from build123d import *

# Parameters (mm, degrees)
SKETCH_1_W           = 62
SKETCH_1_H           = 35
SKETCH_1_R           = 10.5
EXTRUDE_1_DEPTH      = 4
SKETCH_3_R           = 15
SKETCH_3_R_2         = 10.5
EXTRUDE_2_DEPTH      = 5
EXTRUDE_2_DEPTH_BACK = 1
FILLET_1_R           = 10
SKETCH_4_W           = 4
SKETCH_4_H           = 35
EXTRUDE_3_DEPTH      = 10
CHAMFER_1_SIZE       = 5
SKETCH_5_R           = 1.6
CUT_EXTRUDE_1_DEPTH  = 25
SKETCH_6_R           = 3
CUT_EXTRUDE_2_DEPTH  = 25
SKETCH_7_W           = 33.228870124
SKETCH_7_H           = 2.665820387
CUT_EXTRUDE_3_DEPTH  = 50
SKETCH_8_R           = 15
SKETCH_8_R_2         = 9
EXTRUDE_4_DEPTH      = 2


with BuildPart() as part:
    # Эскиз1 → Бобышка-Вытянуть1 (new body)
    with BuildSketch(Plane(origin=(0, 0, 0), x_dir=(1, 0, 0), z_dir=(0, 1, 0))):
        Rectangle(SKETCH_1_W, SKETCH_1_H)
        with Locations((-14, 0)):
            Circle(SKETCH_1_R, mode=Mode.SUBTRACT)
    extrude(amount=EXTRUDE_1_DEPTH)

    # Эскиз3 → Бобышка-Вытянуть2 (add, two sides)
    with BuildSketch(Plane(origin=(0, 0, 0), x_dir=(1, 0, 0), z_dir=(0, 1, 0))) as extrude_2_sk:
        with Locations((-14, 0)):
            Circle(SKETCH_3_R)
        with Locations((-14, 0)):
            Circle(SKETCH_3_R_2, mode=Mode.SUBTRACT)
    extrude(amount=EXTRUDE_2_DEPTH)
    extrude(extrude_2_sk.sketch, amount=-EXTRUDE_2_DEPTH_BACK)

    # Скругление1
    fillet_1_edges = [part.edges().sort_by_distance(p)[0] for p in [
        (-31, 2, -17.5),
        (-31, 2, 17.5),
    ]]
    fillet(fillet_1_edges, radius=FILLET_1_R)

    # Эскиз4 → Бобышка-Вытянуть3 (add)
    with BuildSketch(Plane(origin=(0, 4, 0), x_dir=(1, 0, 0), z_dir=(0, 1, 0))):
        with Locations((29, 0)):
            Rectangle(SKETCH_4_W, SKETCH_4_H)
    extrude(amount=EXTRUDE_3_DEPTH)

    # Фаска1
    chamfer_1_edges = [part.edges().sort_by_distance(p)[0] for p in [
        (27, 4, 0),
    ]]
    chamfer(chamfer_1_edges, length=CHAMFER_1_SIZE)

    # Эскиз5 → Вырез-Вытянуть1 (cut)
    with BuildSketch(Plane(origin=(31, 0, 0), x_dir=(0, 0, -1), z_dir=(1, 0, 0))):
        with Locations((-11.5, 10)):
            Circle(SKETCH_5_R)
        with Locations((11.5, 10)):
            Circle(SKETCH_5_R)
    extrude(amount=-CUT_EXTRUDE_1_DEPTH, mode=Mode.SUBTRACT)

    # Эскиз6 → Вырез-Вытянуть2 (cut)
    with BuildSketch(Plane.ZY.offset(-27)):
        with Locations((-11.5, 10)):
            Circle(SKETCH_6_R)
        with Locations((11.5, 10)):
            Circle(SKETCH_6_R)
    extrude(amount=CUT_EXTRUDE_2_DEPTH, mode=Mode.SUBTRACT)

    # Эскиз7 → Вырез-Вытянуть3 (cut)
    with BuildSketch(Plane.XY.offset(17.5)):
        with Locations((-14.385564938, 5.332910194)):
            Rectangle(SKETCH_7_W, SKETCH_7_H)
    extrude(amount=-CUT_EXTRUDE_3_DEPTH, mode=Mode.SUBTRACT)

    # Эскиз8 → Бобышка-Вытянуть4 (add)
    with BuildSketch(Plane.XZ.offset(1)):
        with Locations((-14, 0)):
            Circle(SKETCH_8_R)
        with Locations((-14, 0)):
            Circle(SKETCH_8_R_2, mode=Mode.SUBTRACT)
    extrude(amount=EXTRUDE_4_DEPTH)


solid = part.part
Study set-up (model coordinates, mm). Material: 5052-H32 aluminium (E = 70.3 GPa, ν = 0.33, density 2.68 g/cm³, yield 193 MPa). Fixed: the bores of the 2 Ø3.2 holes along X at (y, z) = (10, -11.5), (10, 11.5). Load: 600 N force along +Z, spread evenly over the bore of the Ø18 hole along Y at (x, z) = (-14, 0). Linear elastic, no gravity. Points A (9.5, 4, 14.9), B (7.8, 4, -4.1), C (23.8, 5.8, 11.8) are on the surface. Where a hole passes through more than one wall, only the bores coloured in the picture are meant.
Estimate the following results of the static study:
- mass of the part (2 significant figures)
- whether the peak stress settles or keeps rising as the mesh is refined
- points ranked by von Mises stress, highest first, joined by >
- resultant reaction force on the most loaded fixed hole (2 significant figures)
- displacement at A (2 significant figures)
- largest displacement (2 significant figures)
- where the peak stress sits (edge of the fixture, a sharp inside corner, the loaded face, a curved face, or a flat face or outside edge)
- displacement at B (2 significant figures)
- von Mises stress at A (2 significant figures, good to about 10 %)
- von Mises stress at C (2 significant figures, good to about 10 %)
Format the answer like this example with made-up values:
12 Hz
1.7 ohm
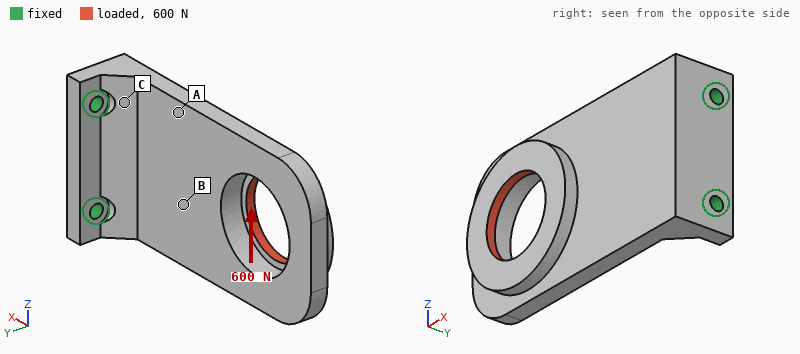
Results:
27 g
keeps rising
C > A > B
1.1 kN
0.035 mm
0.10 mm
edge of the fixture
0.029 mm
23 MPa
42 MPa
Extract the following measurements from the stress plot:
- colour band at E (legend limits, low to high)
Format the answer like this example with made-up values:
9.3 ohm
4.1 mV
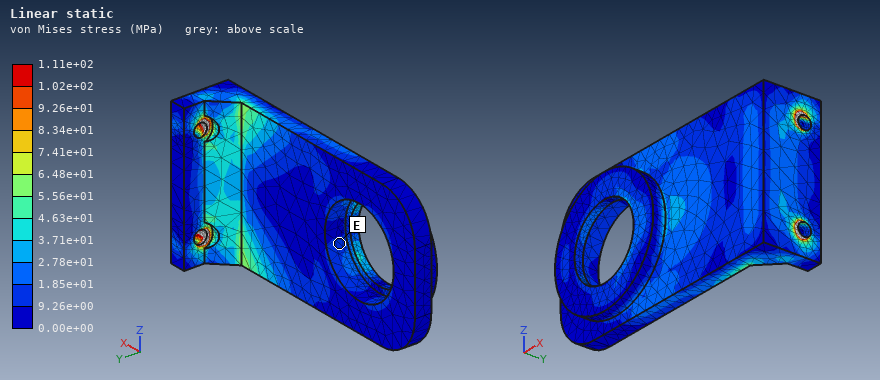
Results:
9.26e+00 to 1.85e+01 MPa
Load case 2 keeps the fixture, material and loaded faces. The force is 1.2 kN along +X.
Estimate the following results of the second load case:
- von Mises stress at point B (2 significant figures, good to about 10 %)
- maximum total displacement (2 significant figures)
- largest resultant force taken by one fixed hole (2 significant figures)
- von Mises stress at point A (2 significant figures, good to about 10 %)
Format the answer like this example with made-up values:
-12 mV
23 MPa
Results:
40 MPa
0.72 mm
600 N
41 MPa
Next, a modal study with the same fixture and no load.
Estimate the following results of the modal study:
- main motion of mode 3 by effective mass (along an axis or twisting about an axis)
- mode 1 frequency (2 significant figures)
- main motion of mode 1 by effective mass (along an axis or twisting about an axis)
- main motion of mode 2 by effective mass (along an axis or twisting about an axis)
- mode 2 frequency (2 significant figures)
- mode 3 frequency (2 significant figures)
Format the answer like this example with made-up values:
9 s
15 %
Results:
along Z
950 Hz
along Y
along Z
3300 Hz
4300 Hz
